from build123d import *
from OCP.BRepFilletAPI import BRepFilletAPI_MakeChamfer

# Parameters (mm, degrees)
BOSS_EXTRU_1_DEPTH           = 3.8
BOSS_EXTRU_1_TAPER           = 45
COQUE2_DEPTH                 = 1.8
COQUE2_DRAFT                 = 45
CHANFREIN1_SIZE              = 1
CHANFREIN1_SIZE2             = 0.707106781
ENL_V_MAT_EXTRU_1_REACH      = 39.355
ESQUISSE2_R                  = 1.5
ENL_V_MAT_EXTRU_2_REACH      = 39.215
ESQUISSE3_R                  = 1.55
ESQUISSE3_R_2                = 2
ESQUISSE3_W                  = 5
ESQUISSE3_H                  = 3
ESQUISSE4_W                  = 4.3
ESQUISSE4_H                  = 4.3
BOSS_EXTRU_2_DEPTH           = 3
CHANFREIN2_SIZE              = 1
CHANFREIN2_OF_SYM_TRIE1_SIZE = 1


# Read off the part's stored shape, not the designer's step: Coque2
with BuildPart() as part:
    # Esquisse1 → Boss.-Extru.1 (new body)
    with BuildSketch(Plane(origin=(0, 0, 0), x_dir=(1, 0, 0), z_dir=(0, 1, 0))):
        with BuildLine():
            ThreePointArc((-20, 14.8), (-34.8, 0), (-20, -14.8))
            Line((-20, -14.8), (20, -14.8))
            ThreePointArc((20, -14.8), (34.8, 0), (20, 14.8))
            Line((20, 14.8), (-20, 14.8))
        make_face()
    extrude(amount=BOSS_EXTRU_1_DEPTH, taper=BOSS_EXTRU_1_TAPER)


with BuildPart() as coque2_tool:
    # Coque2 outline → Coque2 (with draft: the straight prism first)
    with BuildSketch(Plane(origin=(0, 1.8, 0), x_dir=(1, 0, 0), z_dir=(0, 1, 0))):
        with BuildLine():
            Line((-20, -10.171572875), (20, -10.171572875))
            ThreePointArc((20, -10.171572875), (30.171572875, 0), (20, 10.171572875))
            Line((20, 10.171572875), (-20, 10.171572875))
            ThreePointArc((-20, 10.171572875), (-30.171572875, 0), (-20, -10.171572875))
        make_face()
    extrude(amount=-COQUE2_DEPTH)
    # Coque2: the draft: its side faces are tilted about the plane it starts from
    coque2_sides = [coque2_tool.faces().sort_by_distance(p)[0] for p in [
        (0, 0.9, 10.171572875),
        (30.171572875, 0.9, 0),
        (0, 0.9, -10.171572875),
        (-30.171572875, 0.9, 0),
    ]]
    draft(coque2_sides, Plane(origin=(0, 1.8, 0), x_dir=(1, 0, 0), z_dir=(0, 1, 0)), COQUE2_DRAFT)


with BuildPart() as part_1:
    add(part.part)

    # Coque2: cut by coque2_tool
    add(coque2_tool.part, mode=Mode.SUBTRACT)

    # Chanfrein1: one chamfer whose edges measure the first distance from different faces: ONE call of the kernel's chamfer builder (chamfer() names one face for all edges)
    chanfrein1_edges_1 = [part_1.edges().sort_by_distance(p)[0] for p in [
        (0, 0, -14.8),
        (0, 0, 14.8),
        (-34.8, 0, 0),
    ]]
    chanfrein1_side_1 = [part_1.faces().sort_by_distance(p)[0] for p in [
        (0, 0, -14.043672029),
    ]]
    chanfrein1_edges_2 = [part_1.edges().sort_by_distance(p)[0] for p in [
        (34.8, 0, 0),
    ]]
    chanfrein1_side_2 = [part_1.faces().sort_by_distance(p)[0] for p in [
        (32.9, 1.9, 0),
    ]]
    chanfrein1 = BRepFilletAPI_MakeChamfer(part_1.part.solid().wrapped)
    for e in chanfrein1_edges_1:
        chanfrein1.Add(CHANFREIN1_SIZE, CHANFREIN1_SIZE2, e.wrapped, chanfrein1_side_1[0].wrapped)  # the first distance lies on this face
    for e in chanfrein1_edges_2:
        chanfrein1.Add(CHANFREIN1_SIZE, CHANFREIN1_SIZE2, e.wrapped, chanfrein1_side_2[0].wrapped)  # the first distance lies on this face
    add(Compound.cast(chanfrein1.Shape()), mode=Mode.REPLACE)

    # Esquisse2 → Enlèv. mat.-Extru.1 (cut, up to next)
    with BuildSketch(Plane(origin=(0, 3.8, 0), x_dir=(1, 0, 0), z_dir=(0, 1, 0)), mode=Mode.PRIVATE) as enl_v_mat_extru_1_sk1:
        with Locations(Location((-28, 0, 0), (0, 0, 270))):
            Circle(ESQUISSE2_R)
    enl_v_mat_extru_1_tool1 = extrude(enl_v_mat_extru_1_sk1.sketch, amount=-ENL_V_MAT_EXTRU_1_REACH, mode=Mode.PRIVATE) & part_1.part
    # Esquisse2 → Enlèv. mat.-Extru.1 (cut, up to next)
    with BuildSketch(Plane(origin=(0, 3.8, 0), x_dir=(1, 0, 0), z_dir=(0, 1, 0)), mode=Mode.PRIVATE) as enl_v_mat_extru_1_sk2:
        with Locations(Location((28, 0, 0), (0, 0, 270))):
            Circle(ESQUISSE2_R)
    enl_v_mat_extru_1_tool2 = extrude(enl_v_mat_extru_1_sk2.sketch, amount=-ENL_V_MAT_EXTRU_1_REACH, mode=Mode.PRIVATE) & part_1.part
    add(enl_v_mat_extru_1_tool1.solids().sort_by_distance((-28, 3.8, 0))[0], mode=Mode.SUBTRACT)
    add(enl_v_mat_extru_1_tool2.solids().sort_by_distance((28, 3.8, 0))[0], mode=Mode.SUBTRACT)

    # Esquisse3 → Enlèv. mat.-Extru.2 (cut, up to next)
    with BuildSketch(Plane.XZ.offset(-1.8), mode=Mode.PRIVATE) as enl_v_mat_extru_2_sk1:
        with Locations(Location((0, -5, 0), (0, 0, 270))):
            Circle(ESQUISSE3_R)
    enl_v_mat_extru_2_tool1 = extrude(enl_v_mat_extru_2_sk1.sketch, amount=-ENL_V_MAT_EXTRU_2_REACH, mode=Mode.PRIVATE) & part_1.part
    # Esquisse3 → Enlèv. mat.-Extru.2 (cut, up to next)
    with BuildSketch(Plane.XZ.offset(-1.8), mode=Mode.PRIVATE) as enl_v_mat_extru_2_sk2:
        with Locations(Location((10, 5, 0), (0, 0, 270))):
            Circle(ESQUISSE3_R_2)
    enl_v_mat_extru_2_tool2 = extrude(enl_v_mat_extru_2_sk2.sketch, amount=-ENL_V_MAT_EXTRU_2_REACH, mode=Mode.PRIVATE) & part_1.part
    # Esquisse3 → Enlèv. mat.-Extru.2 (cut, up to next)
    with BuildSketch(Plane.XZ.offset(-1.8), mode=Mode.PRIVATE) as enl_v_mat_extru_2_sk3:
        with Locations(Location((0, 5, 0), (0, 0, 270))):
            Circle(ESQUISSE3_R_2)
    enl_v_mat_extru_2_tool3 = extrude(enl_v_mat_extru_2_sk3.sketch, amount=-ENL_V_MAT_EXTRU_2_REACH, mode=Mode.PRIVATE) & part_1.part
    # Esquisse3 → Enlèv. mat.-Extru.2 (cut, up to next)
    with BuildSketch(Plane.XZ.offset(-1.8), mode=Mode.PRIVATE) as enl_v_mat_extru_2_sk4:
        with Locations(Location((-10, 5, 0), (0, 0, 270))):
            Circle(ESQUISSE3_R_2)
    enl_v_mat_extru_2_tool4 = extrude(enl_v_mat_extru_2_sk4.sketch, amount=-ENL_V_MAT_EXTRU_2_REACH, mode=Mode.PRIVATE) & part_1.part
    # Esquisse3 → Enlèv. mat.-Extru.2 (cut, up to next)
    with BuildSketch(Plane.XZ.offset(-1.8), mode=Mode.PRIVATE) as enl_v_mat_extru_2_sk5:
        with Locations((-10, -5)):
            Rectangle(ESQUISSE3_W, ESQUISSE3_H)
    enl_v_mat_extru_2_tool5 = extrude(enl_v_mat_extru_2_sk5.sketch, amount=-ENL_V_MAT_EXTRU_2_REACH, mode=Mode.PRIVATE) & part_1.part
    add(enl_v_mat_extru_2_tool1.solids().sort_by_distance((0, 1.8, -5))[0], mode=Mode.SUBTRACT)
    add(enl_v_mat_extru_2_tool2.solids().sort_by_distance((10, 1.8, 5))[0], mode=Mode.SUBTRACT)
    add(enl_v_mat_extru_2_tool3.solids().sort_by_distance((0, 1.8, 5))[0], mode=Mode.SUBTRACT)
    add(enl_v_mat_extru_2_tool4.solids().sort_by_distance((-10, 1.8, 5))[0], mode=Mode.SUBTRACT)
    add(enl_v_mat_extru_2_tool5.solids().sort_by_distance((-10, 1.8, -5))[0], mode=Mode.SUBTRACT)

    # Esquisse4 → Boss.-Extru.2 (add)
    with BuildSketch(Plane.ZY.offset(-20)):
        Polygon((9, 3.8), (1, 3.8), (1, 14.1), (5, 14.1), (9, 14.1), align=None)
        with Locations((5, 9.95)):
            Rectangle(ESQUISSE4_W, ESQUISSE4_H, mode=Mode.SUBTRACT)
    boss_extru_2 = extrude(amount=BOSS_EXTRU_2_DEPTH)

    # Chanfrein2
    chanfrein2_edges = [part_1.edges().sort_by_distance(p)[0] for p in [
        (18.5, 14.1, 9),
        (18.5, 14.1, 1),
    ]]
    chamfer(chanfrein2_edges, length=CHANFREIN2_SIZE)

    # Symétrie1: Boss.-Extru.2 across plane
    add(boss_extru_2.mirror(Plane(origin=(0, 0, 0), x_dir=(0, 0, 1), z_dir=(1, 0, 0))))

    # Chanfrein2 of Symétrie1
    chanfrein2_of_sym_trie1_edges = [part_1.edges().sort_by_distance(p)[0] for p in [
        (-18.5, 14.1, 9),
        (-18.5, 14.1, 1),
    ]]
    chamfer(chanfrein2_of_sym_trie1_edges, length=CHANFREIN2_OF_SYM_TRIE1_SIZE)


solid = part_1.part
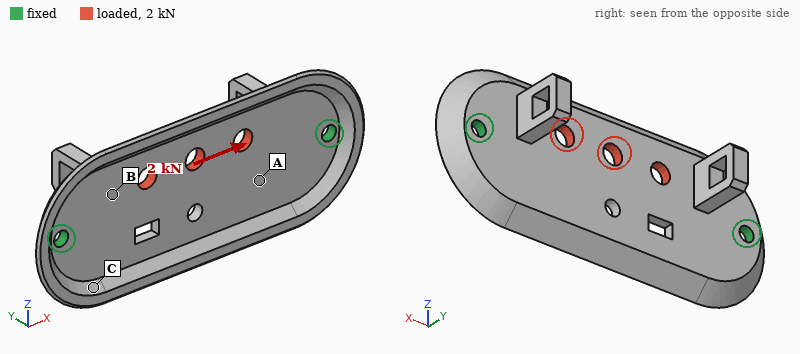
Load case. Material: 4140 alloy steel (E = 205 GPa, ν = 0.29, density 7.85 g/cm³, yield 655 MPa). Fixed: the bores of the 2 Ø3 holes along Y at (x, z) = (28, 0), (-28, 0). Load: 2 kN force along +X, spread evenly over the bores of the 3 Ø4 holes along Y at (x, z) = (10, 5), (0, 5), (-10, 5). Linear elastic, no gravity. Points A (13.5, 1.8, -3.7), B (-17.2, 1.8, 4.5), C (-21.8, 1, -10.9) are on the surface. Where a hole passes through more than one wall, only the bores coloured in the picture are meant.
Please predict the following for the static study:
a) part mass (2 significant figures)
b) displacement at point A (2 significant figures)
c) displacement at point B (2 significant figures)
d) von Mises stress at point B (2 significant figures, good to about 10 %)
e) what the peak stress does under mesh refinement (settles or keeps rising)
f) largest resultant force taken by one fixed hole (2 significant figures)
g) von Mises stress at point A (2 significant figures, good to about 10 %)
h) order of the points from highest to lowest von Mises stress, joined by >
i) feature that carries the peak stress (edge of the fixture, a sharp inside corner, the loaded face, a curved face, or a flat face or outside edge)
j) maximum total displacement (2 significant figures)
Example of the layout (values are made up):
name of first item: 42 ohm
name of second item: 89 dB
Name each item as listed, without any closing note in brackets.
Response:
part mass: 30 g
displacement at point A: 2.4 µm
displacement at point B: 2.6 µm
von Mises stress at point B: 35 MPa
what the peak stress does under mesh refinement: keeps rising
largest resultant force taken by one fixed hole: 1.0 kN
von Mises stress at point A: 19 MPa
order of the points from highest to lowest von Mises stress, joined by >: B > A > C
feature that carries the peak stress: edge of the fixture
maximum total displacement: 4.8 µm
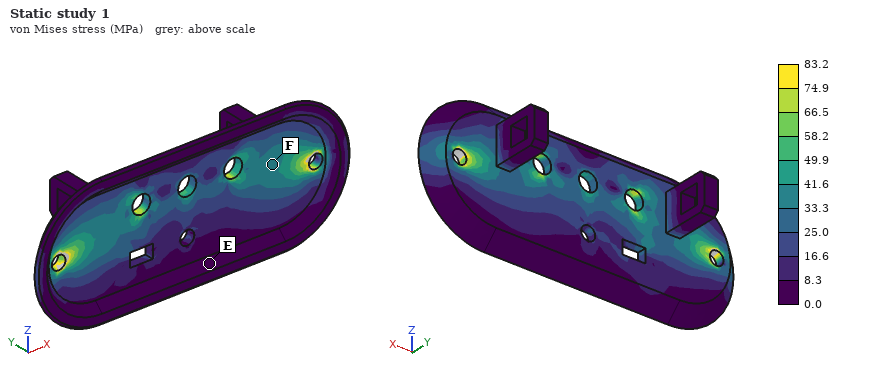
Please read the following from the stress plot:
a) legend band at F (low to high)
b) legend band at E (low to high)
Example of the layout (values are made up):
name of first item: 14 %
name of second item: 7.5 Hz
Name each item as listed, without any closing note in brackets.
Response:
legend band at F: 33.3 to 41.6 MPa
legend band at E: 0.0 to 8.3 MPa
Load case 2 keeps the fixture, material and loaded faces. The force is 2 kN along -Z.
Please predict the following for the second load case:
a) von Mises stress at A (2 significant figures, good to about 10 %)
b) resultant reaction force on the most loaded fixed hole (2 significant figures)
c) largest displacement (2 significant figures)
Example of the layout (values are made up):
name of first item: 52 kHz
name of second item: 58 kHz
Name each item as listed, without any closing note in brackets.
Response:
von Mises stress at A: 60 MPa
resultant reaction force on the most loaded fixed hole: 1.0 kN
largest displacement: 28 µm
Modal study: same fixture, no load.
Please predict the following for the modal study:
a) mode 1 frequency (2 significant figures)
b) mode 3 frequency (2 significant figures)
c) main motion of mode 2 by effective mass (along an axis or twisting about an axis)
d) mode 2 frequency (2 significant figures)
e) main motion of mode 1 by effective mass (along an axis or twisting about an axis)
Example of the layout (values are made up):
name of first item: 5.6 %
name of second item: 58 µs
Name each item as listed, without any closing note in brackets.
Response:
mode 1 frequency: 3500 Hz
mode 3 frequency: 7800 Hz
main motion of mode 2 by effective mass: twisting about X
mode 2 frequency: 4000 Hz
main motion of mode 1 by effective mass: along Y
